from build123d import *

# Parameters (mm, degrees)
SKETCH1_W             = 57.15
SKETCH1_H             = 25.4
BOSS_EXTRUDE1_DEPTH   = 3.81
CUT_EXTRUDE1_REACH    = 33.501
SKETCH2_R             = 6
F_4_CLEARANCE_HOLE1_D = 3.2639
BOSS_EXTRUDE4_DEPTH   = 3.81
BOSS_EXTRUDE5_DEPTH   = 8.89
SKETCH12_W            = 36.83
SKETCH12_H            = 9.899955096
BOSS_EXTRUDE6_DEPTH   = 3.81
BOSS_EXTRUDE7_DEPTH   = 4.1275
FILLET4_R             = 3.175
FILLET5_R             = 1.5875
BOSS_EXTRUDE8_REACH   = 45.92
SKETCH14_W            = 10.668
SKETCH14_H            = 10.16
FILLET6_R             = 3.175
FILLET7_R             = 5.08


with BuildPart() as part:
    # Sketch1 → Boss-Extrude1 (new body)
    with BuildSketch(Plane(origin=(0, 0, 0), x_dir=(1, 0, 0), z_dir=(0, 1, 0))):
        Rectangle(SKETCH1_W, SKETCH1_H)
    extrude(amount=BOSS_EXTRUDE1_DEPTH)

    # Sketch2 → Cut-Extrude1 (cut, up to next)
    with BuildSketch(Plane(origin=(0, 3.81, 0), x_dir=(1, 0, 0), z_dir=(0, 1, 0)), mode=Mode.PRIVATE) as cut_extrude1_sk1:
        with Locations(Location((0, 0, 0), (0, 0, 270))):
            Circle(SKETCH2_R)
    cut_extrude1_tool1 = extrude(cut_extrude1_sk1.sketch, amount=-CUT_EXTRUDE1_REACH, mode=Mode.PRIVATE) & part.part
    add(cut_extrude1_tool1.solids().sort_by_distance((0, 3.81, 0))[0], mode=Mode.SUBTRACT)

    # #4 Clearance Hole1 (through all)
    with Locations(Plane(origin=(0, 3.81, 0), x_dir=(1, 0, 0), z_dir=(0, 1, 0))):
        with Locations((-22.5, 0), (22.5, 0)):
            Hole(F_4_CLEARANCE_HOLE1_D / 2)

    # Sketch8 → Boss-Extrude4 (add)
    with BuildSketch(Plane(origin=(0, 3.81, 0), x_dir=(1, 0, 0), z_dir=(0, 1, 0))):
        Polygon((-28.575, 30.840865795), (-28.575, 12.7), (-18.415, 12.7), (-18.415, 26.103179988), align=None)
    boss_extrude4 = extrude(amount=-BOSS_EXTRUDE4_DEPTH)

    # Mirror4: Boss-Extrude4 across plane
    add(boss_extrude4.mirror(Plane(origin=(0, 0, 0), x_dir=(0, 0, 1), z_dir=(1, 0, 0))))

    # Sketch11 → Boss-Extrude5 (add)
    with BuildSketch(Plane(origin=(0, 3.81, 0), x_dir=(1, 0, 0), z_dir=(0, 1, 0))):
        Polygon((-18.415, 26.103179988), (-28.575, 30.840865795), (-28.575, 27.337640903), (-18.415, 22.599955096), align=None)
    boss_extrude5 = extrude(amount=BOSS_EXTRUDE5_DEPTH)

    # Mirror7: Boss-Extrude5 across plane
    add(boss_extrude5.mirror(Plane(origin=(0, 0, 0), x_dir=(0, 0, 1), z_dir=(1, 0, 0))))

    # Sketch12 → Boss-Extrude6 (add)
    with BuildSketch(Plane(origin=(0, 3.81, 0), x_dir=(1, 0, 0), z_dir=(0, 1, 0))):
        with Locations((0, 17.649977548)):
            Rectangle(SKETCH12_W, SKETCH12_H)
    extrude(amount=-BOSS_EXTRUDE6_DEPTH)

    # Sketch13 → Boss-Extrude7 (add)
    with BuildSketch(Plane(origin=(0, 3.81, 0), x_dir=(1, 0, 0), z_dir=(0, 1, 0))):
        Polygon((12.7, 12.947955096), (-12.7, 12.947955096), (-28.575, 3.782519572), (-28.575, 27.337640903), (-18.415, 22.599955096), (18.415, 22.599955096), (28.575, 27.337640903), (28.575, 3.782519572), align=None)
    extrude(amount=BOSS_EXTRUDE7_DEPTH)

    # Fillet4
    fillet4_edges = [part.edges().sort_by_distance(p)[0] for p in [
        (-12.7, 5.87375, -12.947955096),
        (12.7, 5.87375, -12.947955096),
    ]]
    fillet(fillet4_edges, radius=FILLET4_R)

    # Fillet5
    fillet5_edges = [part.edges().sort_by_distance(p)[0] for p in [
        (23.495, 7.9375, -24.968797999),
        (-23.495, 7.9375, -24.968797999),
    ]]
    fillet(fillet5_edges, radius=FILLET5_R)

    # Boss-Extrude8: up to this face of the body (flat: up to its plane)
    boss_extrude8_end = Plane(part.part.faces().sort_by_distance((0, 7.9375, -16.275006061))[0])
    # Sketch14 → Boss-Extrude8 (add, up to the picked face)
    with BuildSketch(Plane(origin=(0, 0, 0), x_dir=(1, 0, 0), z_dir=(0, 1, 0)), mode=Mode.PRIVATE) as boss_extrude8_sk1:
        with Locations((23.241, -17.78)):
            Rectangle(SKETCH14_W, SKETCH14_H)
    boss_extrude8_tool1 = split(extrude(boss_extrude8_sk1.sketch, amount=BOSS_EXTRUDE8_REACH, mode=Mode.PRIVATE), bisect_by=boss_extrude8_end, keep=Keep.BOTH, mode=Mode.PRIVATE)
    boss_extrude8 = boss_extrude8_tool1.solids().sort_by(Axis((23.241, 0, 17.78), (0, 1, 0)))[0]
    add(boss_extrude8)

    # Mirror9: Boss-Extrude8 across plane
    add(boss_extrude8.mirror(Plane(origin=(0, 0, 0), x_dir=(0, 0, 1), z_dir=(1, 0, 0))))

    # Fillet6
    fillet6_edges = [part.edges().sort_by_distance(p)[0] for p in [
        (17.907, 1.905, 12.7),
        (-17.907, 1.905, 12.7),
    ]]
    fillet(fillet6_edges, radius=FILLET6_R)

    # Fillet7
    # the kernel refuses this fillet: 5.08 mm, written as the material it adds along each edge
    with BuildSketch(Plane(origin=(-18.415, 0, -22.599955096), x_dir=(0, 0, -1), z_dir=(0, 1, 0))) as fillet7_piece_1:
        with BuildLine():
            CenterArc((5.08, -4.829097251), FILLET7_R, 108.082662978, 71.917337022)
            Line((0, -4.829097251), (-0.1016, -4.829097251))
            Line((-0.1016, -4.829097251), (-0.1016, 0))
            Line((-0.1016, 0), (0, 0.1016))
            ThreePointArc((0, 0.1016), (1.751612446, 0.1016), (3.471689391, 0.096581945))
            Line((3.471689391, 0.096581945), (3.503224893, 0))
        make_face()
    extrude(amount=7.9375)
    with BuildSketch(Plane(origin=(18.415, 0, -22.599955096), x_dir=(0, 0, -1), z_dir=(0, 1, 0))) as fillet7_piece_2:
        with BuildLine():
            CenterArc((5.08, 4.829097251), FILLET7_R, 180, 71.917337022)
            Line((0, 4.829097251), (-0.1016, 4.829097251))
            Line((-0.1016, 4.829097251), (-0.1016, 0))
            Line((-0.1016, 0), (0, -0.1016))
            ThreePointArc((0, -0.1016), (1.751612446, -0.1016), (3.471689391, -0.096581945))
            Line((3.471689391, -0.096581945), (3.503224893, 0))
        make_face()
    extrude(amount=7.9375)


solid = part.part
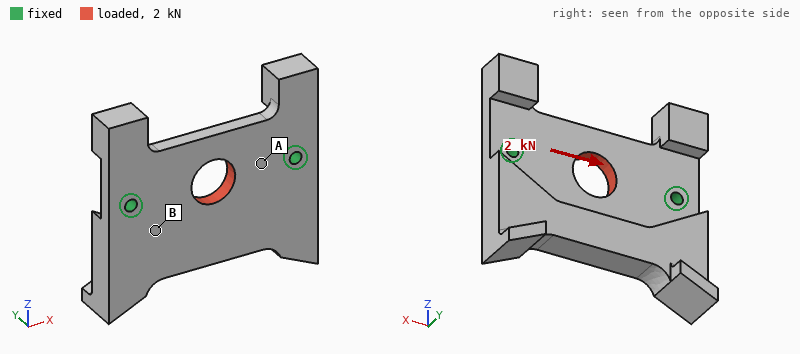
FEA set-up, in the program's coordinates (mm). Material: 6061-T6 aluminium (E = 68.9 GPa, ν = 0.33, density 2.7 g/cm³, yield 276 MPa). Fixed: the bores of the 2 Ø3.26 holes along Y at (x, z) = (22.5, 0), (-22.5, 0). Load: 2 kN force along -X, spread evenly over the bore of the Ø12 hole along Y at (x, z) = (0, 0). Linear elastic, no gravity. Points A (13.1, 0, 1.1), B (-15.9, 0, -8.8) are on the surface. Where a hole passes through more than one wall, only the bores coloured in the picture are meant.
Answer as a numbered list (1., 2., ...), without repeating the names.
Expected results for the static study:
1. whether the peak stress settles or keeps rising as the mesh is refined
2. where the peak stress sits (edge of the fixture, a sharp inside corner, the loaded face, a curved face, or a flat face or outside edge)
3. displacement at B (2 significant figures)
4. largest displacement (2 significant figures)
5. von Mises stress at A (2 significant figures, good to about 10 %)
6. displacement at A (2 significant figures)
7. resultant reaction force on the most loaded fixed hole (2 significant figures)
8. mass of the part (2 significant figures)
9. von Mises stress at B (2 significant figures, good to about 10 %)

1. keeps rising
2. edge of the fixture
3. 2.8 µm
4. 5.7 µm
5. 19 MPa
6. 2.9 µm
7. 1.0 kN
8. 36 g
9. 6.4 MPa
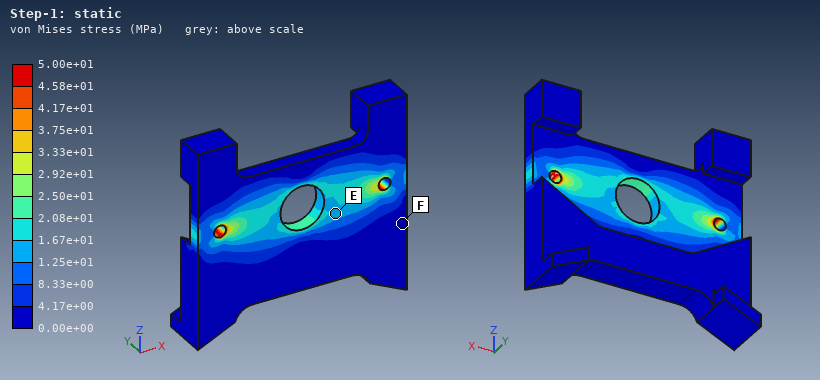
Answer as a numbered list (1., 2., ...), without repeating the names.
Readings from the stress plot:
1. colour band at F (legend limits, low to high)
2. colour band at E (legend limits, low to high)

1. 0.00e+00 to 4.17e+00 MPa
2. 1.25e+01 to 1.67e+01 MPa
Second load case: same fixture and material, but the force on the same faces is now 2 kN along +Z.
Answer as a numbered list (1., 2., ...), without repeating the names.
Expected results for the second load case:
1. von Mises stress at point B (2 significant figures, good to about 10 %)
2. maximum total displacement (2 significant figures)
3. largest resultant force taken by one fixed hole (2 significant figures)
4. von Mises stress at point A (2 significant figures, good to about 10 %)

1. 18 MPa
2. 14 µm
3. 1.0 kN
4. 14 MPa
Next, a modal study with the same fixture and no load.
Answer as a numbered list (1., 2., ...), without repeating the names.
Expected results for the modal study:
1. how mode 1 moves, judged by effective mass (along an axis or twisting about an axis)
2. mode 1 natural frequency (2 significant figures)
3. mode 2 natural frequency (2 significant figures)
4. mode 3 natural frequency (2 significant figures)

1. along Y
2. 2600 Hz
3. 5100 Hz
4. 5100 Hz
